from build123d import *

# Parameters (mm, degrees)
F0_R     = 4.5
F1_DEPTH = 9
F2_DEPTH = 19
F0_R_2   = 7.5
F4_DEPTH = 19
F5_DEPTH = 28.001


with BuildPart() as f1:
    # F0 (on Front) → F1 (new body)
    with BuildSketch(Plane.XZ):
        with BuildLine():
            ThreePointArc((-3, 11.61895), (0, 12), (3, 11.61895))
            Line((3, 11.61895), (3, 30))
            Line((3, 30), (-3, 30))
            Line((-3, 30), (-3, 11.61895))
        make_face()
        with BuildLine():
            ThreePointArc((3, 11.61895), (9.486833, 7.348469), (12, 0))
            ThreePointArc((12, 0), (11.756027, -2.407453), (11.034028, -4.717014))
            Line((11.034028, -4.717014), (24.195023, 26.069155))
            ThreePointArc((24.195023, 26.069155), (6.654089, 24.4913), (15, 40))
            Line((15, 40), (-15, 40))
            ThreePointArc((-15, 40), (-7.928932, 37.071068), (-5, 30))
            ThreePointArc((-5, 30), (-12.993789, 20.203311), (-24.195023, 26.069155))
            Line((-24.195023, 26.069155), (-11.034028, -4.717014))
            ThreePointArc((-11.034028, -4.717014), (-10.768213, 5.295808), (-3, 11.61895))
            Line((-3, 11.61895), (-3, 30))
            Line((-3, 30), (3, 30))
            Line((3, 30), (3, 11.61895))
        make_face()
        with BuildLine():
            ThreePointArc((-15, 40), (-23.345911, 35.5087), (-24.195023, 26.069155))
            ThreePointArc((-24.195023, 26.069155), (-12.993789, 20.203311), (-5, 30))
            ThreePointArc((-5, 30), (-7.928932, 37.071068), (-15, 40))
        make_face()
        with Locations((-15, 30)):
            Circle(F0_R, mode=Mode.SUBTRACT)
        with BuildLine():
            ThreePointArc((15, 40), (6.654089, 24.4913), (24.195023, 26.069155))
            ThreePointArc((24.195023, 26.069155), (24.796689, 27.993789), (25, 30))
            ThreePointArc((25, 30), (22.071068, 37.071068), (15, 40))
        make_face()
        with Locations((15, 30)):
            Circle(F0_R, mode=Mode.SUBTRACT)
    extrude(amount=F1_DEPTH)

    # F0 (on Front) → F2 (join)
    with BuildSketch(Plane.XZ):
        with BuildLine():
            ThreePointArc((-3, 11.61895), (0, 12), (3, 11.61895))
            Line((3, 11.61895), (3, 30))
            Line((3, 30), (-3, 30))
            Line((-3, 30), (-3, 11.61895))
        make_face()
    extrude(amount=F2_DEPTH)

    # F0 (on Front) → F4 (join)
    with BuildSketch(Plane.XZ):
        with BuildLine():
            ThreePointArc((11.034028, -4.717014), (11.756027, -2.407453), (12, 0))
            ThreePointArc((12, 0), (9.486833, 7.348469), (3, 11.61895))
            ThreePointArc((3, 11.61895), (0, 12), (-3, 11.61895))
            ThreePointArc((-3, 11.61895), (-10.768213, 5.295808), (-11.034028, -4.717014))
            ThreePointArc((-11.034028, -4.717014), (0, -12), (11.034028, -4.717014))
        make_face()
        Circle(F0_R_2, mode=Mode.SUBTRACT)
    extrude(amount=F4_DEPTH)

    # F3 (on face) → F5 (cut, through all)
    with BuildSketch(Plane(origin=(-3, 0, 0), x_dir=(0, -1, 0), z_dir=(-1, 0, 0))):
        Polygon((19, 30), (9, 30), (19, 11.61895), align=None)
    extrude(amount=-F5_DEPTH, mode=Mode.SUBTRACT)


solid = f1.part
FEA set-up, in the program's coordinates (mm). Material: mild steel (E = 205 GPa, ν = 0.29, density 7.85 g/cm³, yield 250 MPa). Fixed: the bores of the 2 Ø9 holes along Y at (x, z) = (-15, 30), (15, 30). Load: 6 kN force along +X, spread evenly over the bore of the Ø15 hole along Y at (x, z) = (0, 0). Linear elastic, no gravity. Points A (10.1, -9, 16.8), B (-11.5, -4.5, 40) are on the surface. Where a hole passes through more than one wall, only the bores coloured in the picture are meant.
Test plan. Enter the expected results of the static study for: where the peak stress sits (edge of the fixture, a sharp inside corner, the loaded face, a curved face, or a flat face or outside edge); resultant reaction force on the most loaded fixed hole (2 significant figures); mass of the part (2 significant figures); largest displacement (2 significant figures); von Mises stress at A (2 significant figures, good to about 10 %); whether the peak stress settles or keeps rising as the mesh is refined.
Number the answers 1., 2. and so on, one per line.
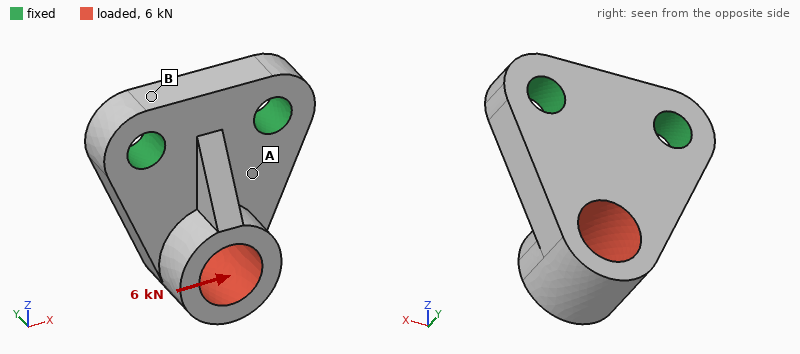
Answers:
1. edge of the fixture
2. 5.9 kN
3. 140 g
4. 26 µm
5. 46 MPa
6. keeps rising
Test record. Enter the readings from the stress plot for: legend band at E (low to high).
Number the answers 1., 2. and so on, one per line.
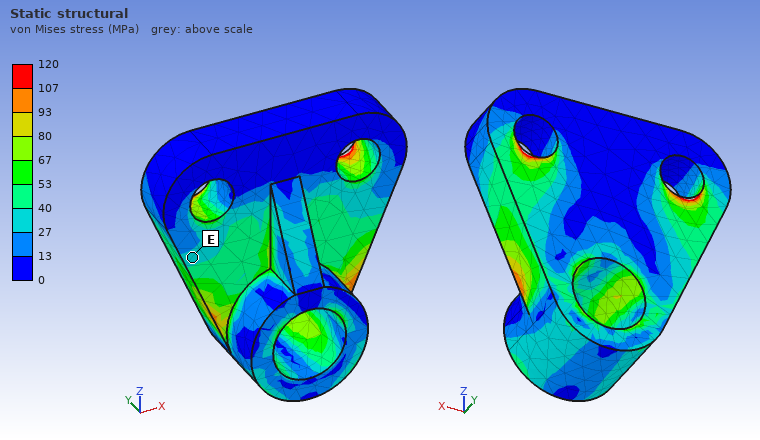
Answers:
1. 27 to 40 MPa
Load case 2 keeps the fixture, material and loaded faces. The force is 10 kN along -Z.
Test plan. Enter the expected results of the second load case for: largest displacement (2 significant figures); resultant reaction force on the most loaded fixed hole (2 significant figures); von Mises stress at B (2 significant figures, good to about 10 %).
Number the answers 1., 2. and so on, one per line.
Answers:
1. 65 µm
2. 5.2 kN
3. 18 MPa
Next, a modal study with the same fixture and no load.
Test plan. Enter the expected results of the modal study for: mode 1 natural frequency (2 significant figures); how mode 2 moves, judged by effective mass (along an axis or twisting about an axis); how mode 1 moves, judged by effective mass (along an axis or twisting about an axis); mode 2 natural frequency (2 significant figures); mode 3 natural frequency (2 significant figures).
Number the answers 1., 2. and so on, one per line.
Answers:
1. 5600 Hz
2. along X
3. along Y
4. 13 kHz
5. 16 kHz
